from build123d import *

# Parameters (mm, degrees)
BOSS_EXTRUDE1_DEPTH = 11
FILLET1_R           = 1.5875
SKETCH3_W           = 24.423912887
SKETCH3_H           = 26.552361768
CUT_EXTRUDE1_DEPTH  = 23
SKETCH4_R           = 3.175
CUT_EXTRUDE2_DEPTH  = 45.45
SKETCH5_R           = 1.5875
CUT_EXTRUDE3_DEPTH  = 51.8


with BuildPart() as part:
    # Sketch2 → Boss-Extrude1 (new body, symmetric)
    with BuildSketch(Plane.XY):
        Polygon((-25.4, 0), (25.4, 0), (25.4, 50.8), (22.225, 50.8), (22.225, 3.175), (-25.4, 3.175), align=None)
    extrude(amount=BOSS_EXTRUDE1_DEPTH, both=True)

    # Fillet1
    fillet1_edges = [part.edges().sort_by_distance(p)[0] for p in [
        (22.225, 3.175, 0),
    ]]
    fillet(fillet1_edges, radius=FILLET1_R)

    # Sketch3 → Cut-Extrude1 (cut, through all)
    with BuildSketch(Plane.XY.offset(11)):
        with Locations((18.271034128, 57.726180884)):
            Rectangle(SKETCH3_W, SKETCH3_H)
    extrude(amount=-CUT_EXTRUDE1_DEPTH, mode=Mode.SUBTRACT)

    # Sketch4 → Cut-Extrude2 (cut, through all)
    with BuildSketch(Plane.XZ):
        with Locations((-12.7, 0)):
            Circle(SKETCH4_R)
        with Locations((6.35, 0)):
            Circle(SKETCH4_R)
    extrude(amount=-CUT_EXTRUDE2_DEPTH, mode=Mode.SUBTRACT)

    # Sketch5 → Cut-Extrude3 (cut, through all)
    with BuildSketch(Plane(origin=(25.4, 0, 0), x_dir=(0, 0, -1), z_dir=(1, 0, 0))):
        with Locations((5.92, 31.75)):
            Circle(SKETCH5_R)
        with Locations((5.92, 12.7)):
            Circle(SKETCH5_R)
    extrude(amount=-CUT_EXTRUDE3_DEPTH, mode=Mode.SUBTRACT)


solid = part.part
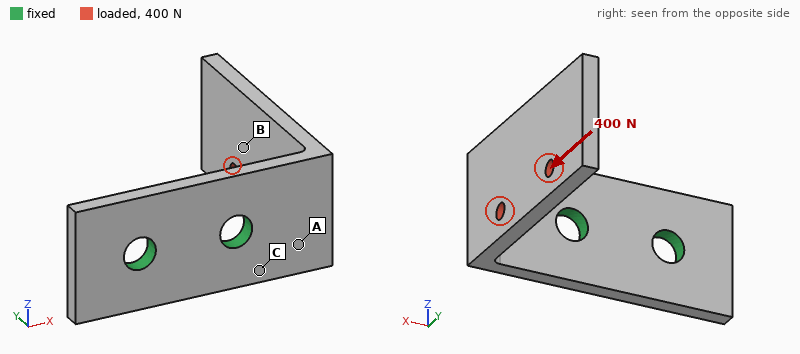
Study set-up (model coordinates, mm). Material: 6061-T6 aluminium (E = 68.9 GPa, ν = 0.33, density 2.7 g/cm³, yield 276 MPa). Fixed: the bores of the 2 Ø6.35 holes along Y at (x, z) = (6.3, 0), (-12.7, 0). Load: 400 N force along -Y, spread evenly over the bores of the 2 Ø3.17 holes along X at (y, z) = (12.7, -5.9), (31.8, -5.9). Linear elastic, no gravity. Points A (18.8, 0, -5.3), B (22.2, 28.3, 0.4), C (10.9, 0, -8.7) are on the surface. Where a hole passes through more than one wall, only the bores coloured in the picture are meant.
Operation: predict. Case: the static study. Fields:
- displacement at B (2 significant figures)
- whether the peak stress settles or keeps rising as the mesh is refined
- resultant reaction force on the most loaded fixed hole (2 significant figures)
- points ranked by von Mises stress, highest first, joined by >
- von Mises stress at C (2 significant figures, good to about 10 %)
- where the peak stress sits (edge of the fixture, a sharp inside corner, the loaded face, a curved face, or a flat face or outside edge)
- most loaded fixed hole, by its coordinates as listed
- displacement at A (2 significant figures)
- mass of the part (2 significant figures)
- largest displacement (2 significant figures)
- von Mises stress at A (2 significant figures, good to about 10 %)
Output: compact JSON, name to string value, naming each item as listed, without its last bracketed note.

{"displacement at B": "0.36 mm", "whether the peak stress settles or keeps rising as the mesh is refined": "keeps rising", "resultant reaction force on the most loaded fixed hole": "440 N", "points ranked by von Mises stress, highest first, joined by >": "C > A > B", "von Mises stress at C": "120 MPa", "where the peak stress sits": "edge of the fixture", "most loaded fixed hole, by its coordinates as listed": "(6.3, 0)", "displacement at A": "0.094 mm", "mass of the part": "17 g", "largest displacement": "0.60 mm", "von Mises stress at A": "52 MPa"}
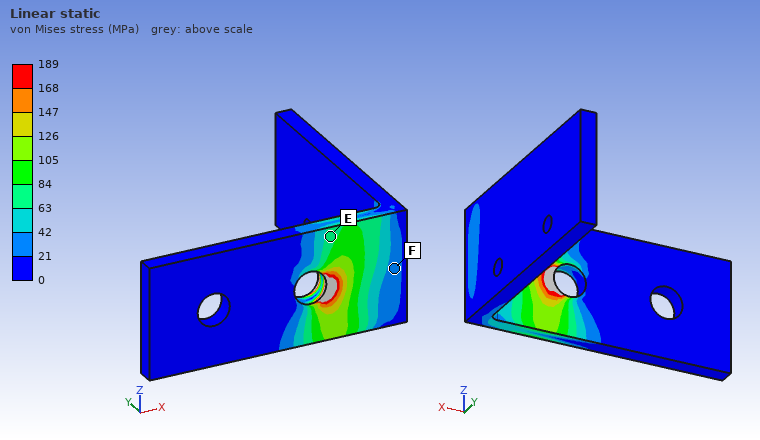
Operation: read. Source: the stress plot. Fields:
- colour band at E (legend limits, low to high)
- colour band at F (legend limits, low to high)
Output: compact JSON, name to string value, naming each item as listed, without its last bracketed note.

{"colour band at E": "63 to 84 MPa", "colour band at F": "21 to 42 MPa"}
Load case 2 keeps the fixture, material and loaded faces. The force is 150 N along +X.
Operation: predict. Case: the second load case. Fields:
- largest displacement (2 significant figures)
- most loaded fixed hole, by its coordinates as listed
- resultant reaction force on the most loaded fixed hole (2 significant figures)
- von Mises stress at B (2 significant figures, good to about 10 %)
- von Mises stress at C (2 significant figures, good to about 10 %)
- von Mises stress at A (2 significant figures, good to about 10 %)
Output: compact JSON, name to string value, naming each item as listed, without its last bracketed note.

{"largest displacement": "0.78 mm", "most loaded fixed hole, by its coordinates as listed": "(6.3, 0)", "resultant reaction force on the most loaded fixed hole": "140 N", "von Mises stress at B": "12 MPa", "von Mises stress at C": "62 MPa", "von Mises stress at A": "76 MPa"}
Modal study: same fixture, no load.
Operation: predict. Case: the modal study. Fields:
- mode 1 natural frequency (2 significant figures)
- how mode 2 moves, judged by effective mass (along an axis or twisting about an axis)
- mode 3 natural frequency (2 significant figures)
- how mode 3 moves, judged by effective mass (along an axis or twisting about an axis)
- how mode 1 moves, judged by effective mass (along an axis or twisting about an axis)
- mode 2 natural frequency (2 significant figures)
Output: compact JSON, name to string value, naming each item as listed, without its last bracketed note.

{"mode 1 natural frequency": "930 Hz", "how mode 2 moves, judged by effective mass": "along Z", "mode 3 natural frequency": "3900 Hz", "how mode 3 moves, judged by effective mass": "along Y", "how mode 1 moves, judged by effective mass": "along X", "mode 2 natural frequency": "1500 Hz"}
